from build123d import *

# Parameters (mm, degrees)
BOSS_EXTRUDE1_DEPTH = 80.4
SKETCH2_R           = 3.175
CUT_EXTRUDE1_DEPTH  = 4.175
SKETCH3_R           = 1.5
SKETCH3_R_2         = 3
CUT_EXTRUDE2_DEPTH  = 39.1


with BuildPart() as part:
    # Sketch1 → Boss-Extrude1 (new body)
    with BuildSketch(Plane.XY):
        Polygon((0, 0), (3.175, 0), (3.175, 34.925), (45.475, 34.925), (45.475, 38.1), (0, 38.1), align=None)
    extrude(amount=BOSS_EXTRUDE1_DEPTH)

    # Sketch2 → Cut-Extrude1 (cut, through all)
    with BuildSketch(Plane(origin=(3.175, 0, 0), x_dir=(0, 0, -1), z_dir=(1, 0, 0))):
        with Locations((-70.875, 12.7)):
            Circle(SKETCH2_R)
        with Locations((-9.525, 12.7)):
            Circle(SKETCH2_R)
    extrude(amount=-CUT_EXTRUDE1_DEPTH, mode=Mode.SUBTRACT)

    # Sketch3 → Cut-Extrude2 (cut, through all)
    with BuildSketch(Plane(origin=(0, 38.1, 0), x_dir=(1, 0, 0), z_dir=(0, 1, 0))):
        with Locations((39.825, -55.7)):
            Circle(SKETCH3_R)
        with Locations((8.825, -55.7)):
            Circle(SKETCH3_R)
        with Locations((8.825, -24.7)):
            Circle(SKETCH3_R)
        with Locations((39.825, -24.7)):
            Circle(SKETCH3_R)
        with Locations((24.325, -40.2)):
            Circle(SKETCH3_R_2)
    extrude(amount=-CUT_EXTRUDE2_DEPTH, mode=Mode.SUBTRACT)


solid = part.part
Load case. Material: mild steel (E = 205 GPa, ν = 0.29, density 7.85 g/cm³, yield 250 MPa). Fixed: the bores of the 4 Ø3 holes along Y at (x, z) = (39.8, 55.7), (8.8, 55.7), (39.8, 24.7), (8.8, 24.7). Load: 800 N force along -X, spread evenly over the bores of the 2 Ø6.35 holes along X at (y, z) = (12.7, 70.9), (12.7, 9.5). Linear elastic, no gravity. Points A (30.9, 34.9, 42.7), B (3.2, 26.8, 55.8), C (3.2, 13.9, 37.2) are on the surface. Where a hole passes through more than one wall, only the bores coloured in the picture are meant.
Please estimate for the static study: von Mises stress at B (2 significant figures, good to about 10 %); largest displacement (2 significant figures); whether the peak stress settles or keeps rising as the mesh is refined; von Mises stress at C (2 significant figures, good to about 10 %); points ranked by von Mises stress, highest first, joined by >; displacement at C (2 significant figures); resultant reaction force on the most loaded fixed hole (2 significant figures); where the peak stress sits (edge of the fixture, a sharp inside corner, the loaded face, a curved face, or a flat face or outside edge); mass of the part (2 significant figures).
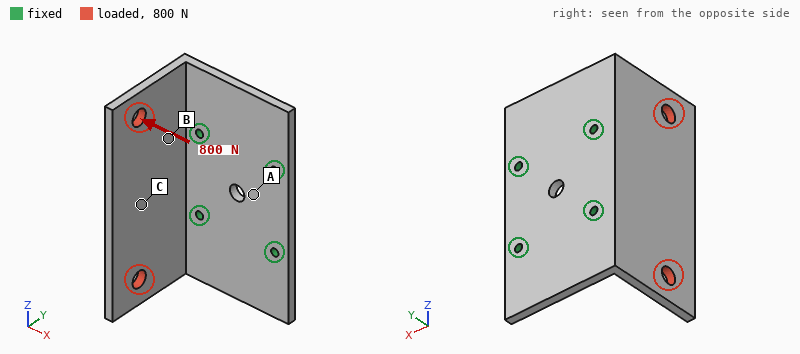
74 MPa
0.31 mm
keeps rising
36 MPa
B > C > A
0.14 mm
310 N
edge of the fixture
160 g
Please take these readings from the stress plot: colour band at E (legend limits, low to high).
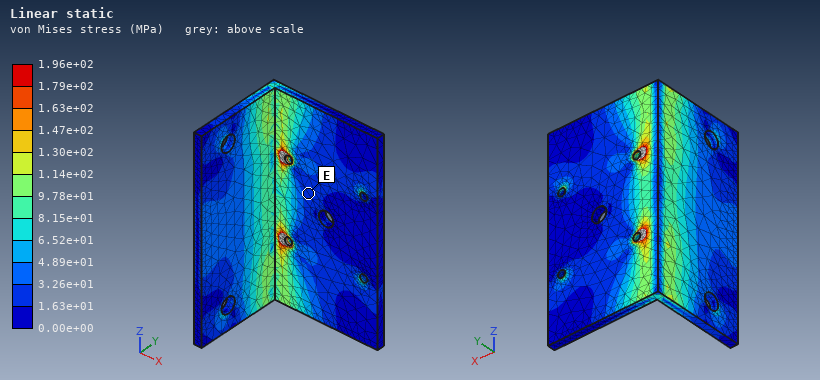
1.63e+01 to 3.26e+01 MPa
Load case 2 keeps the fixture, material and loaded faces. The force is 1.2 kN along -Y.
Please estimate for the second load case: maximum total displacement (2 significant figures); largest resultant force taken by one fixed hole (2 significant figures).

44 µm
670 N
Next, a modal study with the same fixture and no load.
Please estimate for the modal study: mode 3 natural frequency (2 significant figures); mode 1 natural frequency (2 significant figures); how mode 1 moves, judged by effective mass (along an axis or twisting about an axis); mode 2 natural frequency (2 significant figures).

4200 Hz
1400 Hz
along X
2300 Hz
